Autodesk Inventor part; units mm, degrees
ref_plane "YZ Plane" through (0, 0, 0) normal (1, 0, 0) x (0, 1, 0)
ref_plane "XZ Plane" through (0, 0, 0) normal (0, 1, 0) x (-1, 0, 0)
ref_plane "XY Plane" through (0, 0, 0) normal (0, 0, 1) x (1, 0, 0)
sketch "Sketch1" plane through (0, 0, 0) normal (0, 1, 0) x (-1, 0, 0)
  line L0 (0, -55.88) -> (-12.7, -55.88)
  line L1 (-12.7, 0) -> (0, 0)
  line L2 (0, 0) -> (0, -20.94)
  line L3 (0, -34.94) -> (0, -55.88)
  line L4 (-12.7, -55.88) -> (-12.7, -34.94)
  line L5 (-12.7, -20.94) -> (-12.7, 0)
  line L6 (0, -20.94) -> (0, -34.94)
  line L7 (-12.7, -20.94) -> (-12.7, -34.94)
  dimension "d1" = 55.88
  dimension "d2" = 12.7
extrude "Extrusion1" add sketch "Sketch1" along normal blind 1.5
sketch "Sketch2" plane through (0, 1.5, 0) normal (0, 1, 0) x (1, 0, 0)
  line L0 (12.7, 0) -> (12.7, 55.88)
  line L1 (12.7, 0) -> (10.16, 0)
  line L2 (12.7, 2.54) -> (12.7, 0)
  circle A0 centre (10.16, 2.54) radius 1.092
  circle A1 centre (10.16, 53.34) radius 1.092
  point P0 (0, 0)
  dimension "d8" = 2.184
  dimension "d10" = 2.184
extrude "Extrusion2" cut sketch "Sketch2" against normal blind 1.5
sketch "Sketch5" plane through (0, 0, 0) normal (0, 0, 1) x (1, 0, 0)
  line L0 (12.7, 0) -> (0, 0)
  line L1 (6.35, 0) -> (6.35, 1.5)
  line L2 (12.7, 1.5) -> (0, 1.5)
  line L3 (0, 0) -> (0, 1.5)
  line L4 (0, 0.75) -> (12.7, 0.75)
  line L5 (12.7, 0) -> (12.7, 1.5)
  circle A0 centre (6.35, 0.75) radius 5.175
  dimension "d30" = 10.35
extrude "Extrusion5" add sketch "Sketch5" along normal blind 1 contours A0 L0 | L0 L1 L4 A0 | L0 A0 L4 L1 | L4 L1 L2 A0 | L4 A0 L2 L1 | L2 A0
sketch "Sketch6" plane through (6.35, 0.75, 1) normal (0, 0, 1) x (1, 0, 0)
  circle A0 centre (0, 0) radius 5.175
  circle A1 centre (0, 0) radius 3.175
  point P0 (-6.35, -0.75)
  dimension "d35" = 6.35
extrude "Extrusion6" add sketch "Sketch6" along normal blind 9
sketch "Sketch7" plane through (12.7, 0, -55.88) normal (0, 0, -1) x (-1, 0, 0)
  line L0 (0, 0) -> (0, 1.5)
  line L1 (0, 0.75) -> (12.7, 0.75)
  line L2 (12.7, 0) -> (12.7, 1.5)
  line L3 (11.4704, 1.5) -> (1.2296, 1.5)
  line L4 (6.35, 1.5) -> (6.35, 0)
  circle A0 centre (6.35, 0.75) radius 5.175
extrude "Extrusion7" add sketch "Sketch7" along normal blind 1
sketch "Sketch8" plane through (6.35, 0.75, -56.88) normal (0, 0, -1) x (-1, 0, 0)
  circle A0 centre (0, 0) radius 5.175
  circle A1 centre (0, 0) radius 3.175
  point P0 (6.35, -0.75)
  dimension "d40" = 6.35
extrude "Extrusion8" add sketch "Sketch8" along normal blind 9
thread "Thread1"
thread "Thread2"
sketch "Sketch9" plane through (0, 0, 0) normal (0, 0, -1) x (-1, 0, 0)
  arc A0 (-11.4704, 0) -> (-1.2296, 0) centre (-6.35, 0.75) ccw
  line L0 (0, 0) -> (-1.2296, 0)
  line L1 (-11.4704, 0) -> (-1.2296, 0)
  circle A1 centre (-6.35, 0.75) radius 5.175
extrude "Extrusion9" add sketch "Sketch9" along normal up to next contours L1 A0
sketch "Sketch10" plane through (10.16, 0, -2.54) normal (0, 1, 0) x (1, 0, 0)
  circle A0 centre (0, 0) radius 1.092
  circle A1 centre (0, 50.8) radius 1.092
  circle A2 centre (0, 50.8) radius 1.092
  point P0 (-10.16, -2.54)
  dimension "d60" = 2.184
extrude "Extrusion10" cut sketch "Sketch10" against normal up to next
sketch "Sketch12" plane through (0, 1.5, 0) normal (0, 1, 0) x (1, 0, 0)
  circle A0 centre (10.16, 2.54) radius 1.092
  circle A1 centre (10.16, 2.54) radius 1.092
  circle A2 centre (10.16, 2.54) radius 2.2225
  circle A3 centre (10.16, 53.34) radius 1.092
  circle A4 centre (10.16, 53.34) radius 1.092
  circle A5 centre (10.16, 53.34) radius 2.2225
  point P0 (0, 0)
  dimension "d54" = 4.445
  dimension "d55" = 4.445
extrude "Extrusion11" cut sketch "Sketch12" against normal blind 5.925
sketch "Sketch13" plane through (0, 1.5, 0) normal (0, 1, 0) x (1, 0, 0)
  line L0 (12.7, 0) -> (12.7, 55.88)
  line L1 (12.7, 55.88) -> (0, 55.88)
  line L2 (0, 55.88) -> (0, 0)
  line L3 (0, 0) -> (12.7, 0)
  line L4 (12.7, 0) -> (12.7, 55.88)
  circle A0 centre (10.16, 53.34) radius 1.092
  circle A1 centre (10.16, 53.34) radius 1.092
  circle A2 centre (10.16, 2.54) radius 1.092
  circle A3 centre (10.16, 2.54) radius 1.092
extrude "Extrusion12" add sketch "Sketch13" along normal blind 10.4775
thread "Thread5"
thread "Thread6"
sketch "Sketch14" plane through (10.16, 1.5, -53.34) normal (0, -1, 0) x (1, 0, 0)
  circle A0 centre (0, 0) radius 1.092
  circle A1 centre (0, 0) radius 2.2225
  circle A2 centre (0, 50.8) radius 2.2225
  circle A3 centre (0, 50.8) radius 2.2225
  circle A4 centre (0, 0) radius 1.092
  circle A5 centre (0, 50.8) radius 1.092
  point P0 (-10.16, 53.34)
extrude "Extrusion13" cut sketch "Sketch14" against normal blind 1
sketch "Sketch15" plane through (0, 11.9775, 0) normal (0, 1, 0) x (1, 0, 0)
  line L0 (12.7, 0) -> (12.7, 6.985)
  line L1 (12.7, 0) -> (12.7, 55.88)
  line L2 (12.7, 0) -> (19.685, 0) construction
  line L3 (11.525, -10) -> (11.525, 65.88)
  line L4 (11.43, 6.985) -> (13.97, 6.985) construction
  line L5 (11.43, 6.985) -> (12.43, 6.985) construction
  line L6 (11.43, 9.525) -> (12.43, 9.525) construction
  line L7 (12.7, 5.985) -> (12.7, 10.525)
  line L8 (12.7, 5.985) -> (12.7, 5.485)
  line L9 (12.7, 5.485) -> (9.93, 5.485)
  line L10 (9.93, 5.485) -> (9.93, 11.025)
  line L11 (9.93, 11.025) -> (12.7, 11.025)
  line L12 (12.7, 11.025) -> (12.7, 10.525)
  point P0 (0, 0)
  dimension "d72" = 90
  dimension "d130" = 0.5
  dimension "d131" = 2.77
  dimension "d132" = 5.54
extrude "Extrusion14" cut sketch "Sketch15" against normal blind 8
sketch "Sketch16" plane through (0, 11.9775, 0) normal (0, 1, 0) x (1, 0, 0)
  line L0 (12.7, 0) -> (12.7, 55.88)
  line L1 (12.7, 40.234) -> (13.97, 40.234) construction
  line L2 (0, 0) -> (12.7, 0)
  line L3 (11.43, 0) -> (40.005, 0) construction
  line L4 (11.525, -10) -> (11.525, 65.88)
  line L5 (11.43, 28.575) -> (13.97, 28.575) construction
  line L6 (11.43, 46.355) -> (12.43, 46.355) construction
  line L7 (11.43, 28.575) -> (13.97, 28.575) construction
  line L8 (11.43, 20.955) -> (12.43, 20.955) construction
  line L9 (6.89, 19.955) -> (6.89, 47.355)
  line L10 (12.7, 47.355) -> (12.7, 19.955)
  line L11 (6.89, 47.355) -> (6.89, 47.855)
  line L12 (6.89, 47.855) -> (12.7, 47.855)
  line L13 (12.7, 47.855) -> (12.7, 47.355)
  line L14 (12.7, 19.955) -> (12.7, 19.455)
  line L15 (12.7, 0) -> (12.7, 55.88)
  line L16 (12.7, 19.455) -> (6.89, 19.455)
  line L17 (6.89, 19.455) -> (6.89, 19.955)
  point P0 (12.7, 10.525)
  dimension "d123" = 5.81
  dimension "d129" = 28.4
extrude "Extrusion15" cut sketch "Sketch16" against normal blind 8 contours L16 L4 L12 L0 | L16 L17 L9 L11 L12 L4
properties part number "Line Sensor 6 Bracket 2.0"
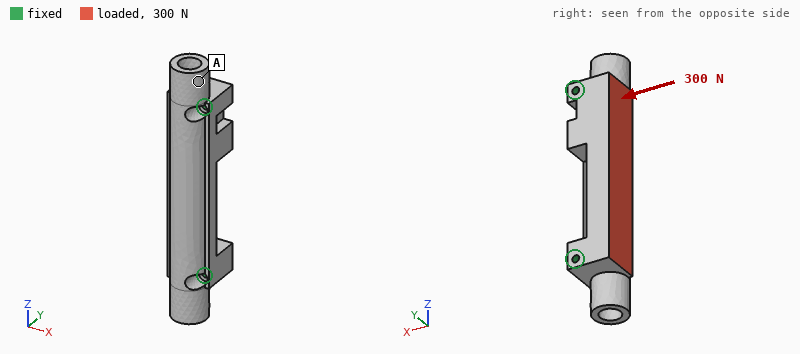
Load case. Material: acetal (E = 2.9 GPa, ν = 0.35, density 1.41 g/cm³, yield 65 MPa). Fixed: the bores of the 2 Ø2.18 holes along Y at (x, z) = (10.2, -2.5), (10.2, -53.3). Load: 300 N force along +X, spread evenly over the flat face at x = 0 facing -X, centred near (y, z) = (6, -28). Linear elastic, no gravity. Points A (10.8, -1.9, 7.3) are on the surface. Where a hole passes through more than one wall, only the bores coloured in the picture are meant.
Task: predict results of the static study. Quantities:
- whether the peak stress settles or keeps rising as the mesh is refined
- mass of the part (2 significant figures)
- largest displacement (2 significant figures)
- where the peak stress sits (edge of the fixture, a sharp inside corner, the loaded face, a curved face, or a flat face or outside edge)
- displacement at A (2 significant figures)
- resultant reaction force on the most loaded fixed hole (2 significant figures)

keeps rising
14 g
70 µm
edge of the fixture
16 µm
200 N
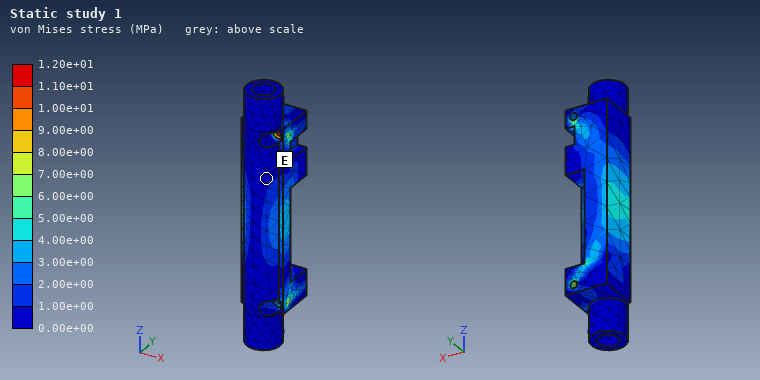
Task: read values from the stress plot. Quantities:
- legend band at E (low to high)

0.00e+00 to 1.00e+00 MPa
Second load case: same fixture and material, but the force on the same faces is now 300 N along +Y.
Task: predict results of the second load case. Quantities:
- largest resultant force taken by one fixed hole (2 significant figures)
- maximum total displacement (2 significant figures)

160 N
0.11 mm
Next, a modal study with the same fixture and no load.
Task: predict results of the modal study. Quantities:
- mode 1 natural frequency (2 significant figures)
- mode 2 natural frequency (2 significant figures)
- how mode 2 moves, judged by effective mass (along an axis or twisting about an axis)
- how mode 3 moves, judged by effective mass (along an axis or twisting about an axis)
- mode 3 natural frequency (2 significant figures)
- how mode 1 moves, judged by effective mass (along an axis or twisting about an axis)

3400 Hz
3900 Hz
along Y
twisting about Z
5100 Hz
along X
